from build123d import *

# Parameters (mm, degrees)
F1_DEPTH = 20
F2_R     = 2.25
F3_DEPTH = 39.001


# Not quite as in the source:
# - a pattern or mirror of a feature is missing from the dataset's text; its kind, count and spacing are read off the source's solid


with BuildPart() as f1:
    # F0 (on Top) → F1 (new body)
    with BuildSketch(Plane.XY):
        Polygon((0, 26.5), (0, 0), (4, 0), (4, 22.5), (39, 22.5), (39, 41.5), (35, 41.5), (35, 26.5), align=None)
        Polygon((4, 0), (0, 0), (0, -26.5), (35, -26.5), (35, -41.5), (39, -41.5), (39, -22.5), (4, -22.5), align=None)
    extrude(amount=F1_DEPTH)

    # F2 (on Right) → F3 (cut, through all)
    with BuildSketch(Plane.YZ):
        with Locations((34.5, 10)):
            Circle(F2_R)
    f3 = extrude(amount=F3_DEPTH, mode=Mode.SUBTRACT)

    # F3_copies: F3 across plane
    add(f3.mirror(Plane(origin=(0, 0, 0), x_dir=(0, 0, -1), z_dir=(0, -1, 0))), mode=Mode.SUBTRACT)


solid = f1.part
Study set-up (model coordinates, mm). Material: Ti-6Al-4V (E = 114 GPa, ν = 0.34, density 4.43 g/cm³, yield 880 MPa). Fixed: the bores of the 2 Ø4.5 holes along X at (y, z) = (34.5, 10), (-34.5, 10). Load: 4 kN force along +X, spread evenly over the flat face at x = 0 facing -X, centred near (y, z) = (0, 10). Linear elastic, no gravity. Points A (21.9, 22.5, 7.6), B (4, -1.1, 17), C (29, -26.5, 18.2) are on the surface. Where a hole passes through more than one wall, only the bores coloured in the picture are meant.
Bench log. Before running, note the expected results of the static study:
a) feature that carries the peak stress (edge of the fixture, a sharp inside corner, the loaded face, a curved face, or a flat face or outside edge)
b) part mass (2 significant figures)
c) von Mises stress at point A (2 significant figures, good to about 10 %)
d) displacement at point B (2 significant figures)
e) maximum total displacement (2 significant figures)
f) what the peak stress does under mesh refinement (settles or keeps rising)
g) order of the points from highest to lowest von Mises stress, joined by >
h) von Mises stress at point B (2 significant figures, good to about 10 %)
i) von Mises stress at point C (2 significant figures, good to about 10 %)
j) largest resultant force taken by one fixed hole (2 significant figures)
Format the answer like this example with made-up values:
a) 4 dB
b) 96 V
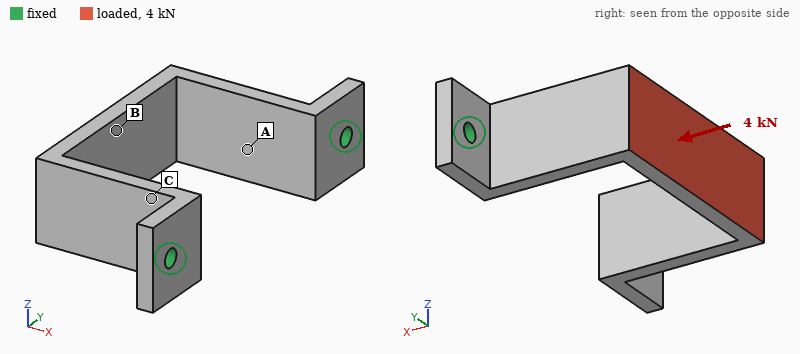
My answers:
a) edge of the fixture
b) 54 g
c) 37 MPa
d) 0.20 mm
e) 0.20 mm
f) keeps rising
g) B > C > A
h) 180 MPa
i) 88 MPa
j) 2.1 kN
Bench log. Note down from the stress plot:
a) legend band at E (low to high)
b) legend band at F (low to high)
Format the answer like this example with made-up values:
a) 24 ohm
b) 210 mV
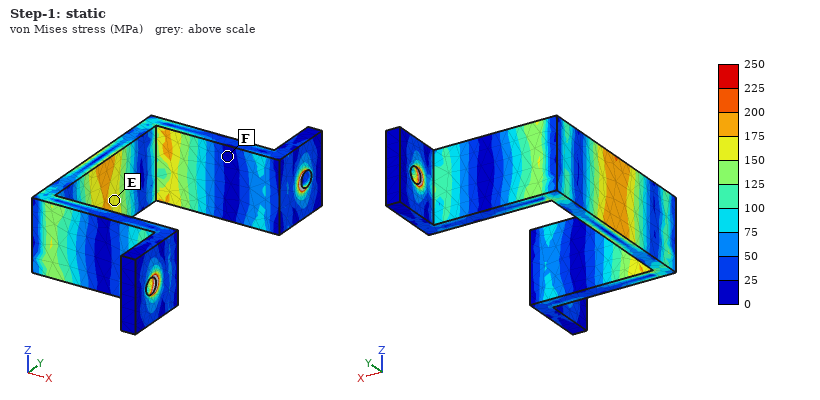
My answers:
a) 150 to 175 MPa
b) 0 to 25 MPa
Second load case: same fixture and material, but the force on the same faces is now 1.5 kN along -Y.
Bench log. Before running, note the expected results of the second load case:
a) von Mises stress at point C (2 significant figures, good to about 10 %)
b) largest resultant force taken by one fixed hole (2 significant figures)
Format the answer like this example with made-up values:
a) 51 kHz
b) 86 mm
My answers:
a) 130 MPa
b) 960 N
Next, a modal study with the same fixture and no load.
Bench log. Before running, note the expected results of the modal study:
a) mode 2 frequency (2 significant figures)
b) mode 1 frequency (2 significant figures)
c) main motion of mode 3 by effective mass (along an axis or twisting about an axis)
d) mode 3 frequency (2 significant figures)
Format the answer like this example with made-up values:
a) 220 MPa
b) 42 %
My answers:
a) 1800 Hz
b) 1800 Hz
c) twisting about X
d) 3000 Hz
